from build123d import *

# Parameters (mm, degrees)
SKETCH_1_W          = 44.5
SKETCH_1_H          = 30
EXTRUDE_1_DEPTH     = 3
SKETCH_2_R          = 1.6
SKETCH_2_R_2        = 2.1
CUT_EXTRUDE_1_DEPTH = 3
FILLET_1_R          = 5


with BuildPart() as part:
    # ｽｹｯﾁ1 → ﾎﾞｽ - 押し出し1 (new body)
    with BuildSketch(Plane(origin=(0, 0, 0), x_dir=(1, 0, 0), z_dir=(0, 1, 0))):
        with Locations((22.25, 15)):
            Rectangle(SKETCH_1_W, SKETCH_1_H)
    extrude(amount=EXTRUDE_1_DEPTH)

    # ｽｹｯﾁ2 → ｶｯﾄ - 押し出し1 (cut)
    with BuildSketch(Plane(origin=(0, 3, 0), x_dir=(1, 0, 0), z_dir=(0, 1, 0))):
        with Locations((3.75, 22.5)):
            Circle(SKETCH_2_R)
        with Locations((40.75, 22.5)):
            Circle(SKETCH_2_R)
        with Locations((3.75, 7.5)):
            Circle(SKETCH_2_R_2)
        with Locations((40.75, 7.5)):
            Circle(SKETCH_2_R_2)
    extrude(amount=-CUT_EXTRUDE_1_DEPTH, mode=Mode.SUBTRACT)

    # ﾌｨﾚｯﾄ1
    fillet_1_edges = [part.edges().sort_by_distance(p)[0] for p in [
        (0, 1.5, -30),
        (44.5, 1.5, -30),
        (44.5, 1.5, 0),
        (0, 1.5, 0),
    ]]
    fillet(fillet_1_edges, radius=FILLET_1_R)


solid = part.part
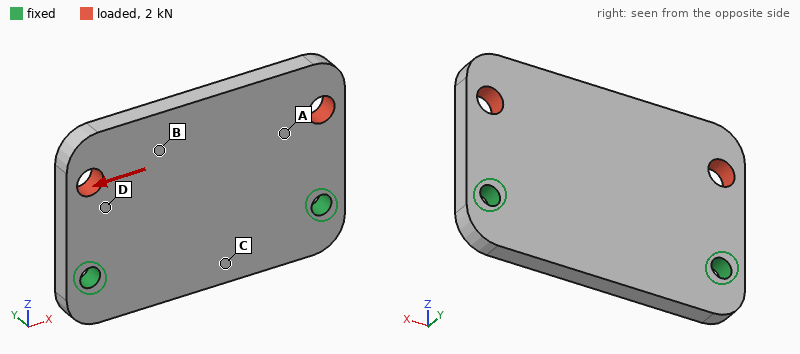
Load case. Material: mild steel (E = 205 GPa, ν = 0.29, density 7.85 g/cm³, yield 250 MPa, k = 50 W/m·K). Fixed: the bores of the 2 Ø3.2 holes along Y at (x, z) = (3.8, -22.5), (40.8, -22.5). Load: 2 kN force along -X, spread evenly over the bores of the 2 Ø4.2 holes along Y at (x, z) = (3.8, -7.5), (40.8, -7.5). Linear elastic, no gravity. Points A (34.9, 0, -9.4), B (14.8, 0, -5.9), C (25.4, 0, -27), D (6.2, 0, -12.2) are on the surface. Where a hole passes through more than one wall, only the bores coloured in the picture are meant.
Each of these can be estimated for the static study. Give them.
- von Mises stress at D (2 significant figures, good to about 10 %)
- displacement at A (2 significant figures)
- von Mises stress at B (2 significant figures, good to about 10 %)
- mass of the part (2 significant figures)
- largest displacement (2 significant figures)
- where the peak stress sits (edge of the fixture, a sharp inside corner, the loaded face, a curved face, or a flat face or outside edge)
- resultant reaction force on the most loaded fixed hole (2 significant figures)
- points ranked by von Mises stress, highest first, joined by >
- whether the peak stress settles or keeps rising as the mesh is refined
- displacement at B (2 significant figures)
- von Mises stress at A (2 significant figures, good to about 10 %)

41 MPa
3.9 µm
18 MPa
30 g
6.7 µm
edge of the fixture
1.3 kN
D > A > B > C
keeps rising
4.2 µm
29 MPa
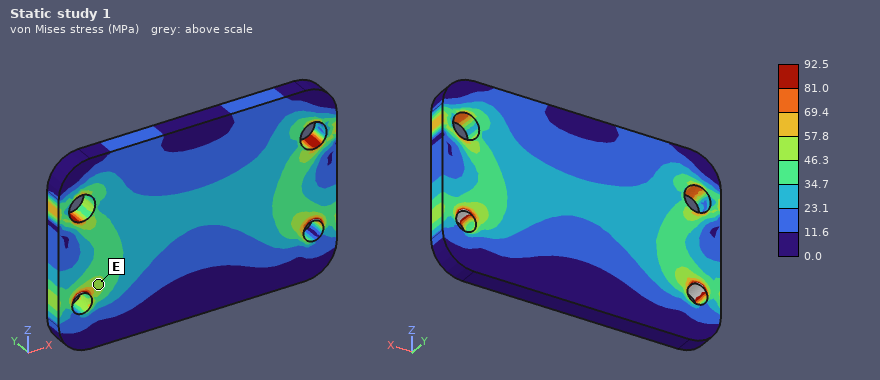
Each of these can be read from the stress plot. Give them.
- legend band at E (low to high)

46.3 to 57.8 MPa
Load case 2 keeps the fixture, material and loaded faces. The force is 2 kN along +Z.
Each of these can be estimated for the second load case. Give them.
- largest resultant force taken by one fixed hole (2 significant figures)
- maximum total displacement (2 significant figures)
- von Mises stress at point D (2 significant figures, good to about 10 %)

1.0 kN
3.6 µm
28 MPa
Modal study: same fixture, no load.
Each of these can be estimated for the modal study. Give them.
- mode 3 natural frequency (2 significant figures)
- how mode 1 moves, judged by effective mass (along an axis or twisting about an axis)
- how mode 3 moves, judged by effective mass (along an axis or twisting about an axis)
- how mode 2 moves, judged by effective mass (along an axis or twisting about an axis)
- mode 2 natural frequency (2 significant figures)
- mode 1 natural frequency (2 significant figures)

11 kHz
along Y
along Y
twisting about Z
8100 Hz
3900 Hz
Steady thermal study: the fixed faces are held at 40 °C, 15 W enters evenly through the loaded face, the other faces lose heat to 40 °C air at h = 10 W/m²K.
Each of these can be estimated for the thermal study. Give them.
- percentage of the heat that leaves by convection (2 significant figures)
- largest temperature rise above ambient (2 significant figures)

5.3 %
62 K
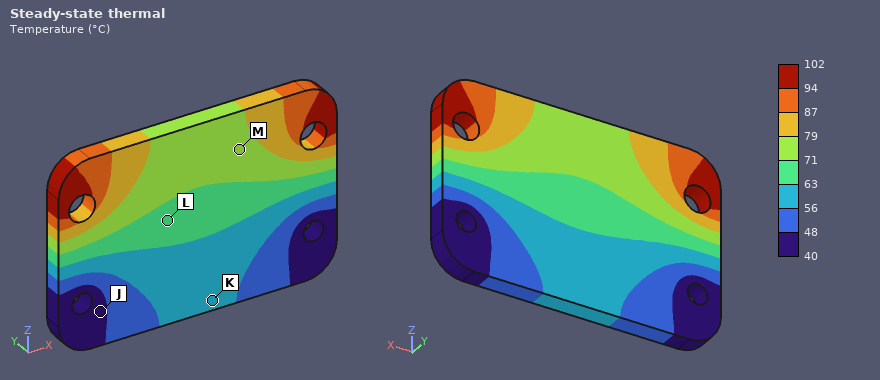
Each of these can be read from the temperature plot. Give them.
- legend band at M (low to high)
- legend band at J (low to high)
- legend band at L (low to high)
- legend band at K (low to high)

71 to 79 °C
40 to 48 °C
63 to 71 °C
56 to 63 °C
